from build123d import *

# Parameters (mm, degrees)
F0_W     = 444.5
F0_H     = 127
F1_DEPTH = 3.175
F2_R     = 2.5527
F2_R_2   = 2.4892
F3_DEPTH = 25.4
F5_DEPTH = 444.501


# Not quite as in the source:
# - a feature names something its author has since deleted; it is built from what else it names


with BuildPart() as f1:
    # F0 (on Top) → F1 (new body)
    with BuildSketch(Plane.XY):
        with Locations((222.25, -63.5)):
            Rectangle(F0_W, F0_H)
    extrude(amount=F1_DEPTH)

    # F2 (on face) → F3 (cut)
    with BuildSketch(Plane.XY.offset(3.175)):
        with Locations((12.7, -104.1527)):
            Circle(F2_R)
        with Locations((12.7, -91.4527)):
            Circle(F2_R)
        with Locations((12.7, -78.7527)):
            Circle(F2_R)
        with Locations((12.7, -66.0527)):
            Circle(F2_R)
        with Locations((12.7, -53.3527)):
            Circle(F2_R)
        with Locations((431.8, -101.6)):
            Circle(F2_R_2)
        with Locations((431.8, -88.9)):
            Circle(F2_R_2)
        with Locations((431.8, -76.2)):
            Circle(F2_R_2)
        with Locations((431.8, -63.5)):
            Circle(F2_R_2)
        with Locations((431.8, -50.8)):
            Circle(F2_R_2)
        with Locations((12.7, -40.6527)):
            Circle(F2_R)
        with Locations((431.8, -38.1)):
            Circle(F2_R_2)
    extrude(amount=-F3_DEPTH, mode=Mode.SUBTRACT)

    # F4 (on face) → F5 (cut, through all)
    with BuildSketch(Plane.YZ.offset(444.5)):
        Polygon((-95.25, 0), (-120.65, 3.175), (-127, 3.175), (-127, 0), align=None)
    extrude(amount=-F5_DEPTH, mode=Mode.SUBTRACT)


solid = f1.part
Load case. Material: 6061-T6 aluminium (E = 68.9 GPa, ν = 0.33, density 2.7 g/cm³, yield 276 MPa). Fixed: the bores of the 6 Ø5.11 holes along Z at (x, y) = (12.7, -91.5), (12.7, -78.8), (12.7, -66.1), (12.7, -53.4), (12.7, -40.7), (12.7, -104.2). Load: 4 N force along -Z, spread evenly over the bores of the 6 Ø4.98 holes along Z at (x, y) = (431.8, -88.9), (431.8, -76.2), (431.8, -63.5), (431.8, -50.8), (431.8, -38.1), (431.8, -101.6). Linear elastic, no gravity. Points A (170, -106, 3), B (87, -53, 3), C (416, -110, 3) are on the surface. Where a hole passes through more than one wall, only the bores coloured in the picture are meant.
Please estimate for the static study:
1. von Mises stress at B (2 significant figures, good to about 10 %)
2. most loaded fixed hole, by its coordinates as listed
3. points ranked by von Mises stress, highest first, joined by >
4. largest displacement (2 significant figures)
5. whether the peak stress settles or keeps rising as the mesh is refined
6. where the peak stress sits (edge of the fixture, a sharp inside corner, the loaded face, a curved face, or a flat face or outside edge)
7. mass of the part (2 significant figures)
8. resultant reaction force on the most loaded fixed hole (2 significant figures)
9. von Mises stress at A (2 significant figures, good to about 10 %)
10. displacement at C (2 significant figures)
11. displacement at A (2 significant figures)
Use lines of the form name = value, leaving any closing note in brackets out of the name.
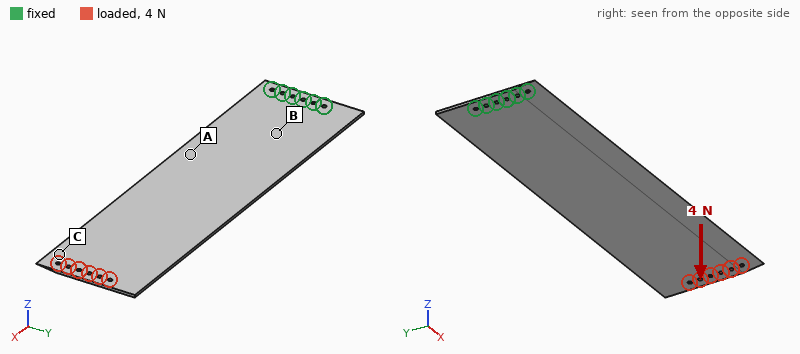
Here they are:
von Mises stress at B = 7.1 MPa
most loaded fixed hole, by its coordinates as listed = (12.7, -104.2)
points ranked by von Mises stress, highest first, joined by > = B > A > C
largest displacement = 5.3 mm
whether the peak stress settles or keeps rising as the mesh is refined = keeps rising
where the peak stress sits = edge of the fixture
mass of the part = 410 g
resultant reaction force on the most loaded fixed hole = 56 N
von Mises stress at A = 5.1 MPa
displacement at C = 4.7 mm
displacement at A = 0.90 mm
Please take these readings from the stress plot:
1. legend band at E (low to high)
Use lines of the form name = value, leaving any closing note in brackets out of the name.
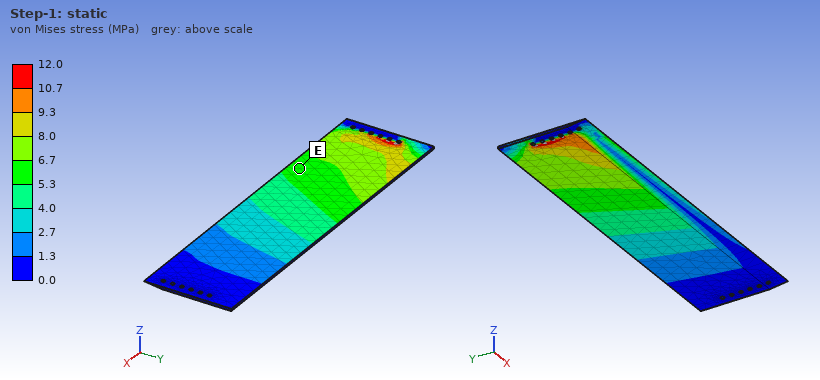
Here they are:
legend band at E = 5.3 to 6.7 MPa
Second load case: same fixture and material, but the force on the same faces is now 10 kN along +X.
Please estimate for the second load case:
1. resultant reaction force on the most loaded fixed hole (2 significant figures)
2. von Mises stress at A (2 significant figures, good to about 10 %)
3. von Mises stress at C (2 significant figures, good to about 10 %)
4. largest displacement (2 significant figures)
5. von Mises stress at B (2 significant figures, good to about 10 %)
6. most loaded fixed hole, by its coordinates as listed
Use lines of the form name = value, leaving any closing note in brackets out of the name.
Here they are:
resultant reaction force on the most loaded fixed hole = 2.7 kN
von Mises stress at A = 48 MPa
von Mises stress at C = 32 MPa
largest displacement = 2.6 mm
von Mises stress at B = 28 MPa
most loaded fixed hole, by its coordinates as listed = (12.7, -40.7)
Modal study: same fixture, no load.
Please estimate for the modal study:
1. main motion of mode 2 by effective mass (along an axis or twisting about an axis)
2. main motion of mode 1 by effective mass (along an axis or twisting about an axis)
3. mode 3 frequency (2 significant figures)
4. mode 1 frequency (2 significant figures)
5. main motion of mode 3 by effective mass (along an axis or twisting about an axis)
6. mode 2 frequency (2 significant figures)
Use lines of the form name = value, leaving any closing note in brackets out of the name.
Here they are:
main motion of mode 2 by effective mass = along Z
main motion of mode 1 by effective mass = along Z
mode 3 frequency = 110 Hz
mode 1 frequency = 14 Hz
main motion of mode 3 by effective mass = twisting about X
mode 2 frequency = 87 Hz
